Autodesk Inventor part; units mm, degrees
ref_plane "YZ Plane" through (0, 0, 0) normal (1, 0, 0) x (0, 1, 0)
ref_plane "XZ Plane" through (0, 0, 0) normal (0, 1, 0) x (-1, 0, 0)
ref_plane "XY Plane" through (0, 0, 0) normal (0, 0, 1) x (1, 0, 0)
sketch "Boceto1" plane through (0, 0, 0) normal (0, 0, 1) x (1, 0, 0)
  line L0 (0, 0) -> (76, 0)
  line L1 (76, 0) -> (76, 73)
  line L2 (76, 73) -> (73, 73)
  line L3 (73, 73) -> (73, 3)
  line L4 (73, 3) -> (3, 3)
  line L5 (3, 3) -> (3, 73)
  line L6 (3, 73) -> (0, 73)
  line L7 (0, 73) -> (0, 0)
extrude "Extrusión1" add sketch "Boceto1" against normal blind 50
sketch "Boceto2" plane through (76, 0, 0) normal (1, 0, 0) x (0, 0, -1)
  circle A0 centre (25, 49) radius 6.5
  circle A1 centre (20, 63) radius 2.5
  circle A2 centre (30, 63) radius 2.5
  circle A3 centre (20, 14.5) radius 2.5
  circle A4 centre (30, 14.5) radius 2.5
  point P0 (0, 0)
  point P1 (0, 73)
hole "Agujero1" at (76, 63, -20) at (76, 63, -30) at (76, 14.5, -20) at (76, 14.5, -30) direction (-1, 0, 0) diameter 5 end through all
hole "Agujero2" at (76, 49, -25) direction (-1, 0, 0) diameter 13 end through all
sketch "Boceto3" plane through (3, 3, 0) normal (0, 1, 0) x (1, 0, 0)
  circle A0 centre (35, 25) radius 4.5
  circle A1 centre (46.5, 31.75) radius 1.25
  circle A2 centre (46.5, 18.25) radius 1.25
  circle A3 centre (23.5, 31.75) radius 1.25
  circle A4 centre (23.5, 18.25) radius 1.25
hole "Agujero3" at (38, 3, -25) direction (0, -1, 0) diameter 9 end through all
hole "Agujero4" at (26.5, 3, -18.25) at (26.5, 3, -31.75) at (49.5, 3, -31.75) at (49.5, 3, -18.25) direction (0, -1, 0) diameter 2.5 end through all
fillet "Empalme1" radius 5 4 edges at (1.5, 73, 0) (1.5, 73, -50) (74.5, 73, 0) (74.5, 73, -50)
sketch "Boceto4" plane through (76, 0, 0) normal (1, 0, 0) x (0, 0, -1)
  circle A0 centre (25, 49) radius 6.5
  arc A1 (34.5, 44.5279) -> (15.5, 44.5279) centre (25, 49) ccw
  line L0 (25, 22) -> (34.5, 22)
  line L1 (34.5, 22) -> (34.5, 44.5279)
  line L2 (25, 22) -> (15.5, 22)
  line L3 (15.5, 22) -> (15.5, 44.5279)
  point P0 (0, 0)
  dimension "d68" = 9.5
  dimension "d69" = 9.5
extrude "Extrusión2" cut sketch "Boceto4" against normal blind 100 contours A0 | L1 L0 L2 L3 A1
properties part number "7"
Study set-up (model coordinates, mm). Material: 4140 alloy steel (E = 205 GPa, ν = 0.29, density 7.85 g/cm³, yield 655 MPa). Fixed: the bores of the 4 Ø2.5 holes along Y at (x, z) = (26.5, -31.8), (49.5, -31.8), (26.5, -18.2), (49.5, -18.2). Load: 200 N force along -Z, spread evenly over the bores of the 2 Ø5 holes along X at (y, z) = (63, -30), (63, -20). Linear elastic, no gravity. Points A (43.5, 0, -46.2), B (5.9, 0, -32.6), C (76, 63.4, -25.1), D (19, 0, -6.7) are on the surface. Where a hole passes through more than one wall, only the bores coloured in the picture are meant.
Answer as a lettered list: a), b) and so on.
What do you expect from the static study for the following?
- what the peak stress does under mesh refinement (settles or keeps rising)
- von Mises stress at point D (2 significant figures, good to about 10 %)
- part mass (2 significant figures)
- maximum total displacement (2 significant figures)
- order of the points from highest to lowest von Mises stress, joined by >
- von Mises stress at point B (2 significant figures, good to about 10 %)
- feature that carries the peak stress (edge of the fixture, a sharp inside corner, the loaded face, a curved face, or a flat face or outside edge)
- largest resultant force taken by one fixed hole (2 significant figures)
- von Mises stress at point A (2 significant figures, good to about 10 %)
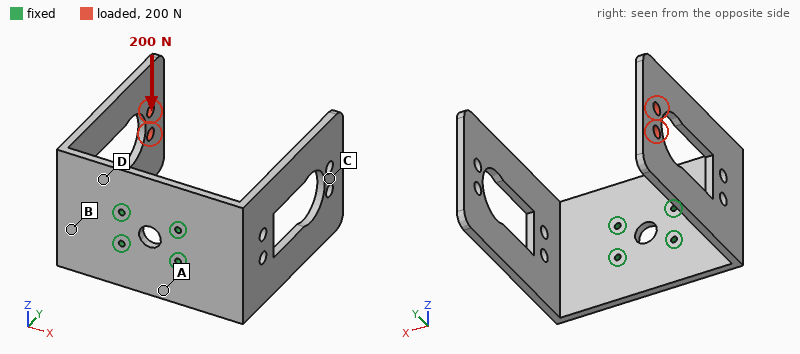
a) keeps rising
b) 64 MPa
c) 220 g
d) 0.43 mm
e) B > D > A > C
f) 79 MPa
g) edge of the fixture
h) 670 N
i) 27 MPa
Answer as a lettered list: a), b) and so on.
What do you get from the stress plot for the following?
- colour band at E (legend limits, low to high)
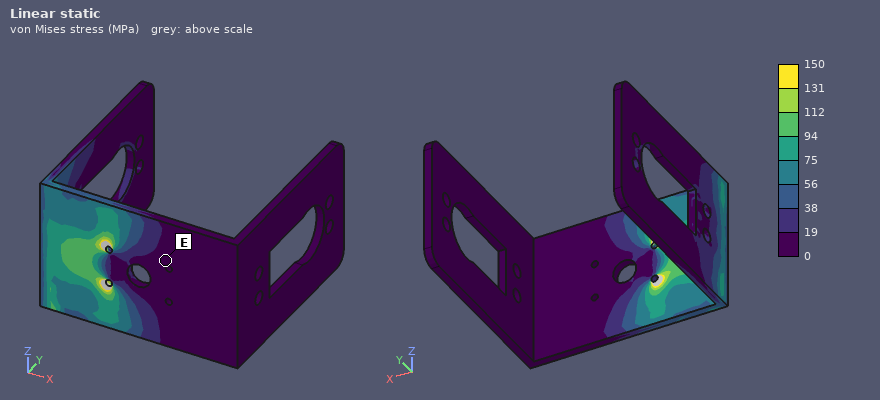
a) 0 to 19 MPa
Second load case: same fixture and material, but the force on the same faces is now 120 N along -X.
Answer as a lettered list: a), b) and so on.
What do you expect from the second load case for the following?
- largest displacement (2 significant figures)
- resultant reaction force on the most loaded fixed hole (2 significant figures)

a) 1.2 mm
b) 87 N
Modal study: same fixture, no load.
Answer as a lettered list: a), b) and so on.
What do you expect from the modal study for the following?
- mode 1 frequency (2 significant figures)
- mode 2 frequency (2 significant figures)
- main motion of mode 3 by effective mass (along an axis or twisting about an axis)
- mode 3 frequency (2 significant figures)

a) 330 Hz
b) 330 Hz
c) twisting about Y
d) 640 Hz
